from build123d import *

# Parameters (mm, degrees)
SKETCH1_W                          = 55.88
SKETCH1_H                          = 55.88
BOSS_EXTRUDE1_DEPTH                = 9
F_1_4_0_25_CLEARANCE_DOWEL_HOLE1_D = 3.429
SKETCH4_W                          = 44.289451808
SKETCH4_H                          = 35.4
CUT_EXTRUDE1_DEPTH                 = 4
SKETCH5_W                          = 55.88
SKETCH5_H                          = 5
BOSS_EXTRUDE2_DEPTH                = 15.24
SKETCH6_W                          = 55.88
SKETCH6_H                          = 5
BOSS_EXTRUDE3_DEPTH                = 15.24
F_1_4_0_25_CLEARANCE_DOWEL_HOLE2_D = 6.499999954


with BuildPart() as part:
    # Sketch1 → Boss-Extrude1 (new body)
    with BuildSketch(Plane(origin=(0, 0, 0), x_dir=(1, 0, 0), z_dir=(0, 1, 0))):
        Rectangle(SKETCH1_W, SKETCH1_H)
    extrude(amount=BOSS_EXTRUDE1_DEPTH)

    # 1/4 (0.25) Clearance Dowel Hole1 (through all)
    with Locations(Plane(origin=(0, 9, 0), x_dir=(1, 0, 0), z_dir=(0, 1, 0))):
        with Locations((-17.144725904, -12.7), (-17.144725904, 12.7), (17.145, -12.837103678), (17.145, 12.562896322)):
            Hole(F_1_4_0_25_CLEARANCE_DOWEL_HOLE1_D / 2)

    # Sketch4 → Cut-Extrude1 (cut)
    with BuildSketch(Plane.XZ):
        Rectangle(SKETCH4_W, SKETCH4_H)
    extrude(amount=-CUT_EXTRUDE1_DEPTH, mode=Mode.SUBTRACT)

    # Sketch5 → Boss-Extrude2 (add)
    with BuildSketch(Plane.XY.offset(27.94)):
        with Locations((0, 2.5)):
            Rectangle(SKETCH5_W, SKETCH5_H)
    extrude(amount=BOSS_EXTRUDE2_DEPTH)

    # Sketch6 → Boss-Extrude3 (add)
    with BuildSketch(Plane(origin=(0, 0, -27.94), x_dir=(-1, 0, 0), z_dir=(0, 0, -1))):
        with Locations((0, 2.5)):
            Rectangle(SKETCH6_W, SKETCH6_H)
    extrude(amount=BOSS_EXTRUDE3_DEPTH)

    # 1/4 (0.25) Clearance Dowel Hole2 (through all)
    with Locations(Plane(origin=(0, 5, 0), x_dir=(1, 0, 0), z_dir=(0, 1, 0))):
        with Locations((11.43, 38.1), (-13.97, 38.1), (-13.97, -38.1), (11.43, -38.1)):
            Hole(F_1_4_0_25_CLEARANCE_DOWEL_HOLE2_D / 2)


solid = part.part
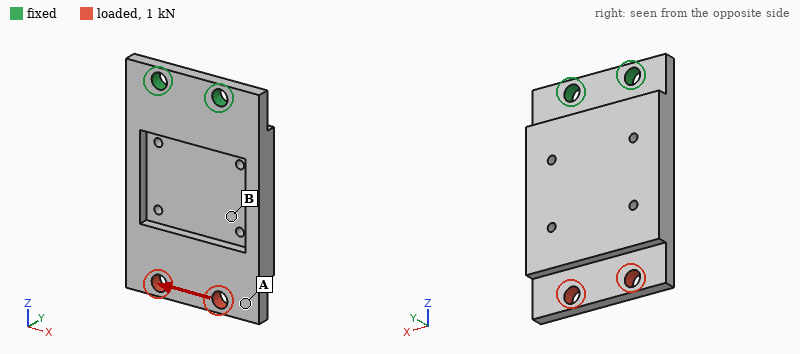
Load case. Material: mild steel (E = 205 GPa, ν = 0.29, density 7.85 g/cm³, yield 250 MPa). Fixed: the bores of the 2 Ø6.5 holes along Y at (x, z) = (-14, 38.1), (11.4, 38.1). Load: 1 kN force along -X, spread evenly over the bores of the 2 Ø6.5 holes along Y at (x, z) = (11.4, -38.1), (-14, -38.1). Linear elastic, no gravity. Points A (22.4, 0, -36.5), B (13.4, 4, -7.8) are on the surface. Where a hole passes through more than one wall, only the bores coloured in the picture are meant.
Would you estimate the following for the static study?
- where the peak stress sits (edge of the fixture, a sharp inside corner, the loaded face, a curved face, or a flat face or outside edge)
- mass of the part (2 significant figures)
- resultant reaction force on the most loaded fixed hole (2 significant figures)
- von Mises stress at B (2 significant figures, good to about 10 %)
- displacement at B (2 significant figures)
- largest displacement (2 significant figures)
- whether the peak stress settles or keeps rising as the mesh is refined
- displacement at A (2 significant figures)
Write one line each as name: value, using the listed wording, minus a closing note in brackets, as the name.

where the peak stress sits: edge of the fixture
mass of the part: 230 g
resultant reaction force on the most loaded fixed hole: 2.5 kN
von Mises stress at B: 17 MPa
displacement at B: 17 µm
largest displacement: 41 µm
whether the peak stress settles or keeps rising as the mesh is refined: keeps rising
displacement at A: 36 µm
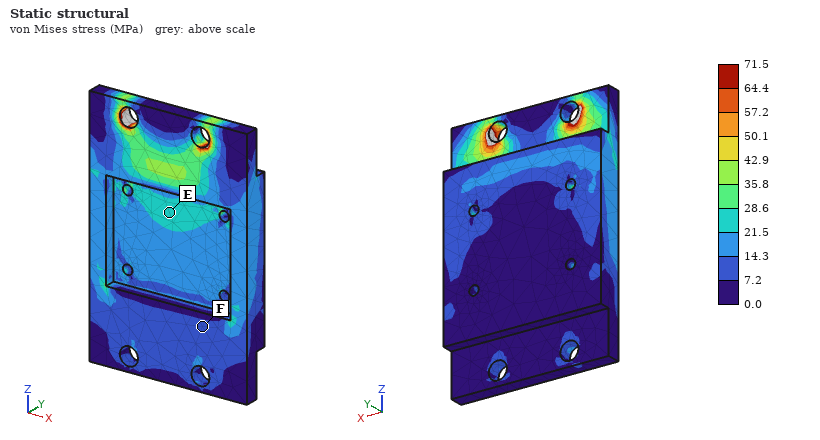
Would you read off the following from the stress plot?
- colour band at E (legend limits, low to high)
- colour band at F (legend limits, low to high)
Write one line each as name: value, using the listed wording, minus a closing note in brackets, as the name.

colour band at E: 21.5 to 28.6 MPa
colour band at F: 7.2 to 14.3 MPa
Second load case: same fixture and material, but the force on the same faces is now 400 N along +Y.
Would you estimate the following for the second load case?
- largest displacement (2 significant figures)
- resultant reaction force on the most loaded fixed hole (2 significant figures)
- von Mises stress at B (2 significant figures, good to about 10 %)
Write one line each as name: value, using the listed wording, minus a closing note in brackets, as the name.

largest displacement: 0.33 mm
resultant reaction force on the most loaded fixed hole: 360 N
von Mises stress at B: 19 MPa
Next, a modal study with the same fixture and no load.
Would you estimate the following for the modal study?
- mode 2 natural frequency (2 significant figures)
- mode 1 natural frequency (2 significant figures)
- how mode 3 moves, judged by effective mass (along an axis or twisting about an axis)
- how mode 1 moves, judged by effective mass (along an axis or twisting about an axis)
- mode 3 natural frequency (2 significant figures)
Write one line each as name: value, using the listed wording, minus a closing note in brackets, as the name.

mode 2 natural frequency: 2200 Hz
mode 1 natural frequency: 720 Hz
how mode 3 moves, judged by effective mass: along X
how mode 1 moves, judged by effective mass: along Y
mode 3 natural frequency: 4100 Hz
